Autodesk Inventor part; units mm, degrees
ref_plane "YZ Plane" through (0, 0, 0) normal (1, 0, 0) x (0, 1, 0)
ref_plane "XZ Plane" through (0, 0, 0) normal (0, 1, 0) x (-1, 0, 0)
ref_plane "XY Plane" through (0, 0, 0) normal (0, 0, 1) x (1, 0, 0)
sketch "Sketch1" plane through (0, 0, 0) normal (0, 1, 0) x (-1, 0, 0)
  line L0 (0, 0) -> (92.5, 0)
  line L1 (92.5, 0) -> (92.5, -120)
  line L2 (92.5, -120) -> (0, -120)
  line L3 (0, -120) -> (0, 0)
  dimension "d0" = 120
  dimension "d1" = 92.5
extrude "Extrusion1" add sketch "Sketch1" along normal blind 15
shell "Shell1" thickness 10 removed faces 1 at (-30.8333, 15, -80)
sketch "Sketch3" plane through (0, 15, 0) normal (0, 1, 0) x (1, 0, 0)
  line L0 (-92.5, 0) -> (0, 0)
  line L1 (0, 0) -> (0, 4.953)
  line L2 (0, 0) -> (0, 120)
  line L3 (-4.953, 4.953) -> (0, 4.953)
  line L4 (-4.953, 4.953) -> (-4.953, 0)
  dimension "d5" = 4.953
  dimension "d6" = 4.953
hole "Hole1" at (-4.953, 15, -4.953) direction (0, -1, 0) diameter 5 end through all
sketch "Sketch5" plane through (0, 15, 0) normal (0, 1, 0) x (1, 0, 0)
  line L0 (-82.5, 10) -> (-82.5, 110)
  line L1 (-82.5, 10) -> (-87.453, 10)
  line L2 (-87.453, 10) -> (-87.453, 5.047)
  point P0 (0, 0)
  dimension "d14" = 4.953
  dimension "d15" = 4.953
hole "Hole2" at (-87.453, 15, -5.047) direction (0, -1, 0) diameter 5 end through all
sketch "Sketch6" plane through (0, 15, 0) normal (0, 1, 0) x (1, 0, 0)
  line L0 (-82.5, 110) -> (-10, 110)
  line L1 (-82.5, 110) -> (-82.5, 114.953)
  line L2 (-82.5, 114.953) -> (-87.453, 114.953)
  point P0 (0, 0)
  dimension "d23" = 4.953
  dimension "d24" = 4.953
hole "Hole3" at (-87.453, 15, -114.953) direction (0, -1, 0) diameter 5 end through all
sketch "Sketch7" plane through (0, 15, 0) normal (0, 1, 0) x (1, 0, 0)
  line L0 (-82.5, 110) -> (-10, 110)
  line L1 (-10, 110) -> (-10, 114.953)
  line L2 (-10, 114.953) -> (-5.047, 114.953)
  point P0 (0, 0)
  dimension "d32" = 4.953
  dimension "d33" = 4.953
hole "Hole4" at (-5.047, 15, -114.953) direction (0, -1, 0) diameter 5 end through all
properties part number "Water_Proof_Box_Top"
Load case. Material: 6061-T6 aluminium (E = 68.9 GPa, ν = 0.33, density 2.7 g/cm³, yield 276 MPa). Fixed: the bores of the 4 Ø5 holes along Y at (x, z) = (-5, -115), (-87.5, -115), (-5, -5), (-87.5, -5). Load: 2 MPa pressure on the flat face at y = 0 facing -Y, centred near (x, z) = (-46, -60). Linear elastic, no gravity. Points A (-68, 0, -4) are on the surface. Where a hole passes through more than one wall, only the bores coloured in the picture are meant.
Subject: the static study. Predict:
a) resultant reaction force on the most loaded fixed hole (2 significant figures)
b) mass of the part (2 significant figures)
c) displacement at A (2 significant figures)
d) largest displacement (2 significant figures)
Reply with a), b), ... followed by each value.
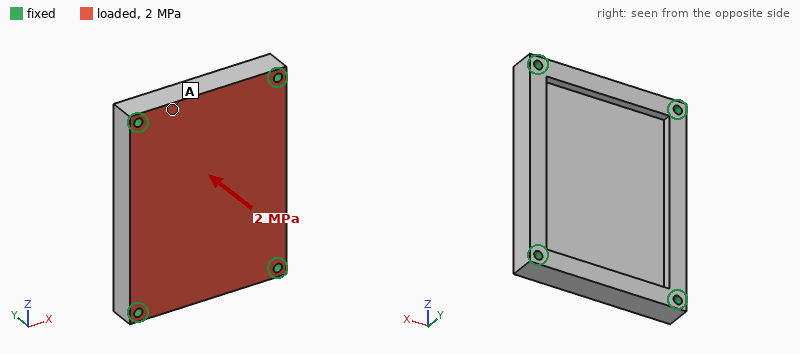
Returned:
a) 5.9 kN
b) 350 g
c) 0.027 mm
d) 0.17 mm
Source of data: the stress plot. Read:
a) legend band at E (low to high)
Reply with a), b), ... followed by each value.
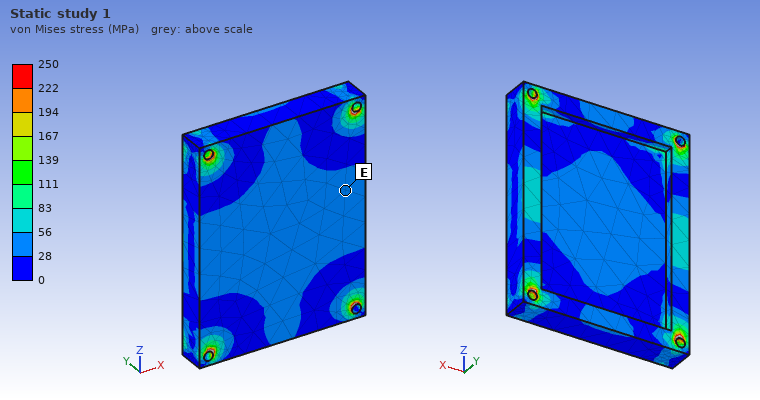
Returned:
a) 28 to 56 MPa
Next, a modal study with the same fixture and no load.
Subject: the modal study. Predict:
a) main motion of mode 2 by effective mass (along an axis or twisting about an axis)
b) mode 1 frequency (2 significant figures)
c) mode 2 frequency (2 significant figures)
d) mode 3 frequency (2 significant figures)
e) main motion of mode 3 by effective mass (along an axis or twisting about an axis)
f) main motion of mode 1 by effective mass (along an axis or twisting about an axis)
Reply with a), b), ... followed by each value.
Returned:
a) twisting about Z
b) 3900 Hz
c) 5900 Hz
d) 8000 Hz
e) twisting about X
f) along Y
